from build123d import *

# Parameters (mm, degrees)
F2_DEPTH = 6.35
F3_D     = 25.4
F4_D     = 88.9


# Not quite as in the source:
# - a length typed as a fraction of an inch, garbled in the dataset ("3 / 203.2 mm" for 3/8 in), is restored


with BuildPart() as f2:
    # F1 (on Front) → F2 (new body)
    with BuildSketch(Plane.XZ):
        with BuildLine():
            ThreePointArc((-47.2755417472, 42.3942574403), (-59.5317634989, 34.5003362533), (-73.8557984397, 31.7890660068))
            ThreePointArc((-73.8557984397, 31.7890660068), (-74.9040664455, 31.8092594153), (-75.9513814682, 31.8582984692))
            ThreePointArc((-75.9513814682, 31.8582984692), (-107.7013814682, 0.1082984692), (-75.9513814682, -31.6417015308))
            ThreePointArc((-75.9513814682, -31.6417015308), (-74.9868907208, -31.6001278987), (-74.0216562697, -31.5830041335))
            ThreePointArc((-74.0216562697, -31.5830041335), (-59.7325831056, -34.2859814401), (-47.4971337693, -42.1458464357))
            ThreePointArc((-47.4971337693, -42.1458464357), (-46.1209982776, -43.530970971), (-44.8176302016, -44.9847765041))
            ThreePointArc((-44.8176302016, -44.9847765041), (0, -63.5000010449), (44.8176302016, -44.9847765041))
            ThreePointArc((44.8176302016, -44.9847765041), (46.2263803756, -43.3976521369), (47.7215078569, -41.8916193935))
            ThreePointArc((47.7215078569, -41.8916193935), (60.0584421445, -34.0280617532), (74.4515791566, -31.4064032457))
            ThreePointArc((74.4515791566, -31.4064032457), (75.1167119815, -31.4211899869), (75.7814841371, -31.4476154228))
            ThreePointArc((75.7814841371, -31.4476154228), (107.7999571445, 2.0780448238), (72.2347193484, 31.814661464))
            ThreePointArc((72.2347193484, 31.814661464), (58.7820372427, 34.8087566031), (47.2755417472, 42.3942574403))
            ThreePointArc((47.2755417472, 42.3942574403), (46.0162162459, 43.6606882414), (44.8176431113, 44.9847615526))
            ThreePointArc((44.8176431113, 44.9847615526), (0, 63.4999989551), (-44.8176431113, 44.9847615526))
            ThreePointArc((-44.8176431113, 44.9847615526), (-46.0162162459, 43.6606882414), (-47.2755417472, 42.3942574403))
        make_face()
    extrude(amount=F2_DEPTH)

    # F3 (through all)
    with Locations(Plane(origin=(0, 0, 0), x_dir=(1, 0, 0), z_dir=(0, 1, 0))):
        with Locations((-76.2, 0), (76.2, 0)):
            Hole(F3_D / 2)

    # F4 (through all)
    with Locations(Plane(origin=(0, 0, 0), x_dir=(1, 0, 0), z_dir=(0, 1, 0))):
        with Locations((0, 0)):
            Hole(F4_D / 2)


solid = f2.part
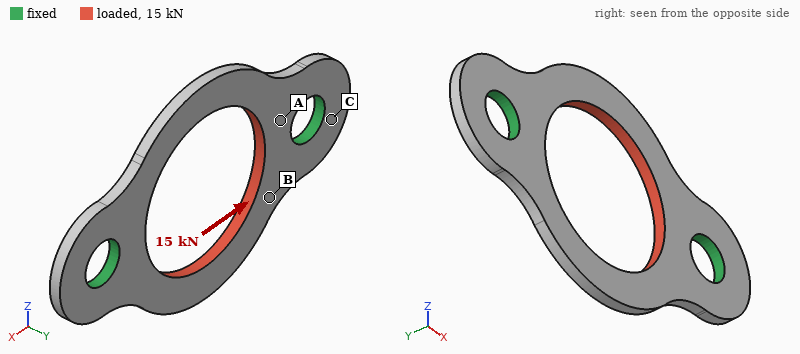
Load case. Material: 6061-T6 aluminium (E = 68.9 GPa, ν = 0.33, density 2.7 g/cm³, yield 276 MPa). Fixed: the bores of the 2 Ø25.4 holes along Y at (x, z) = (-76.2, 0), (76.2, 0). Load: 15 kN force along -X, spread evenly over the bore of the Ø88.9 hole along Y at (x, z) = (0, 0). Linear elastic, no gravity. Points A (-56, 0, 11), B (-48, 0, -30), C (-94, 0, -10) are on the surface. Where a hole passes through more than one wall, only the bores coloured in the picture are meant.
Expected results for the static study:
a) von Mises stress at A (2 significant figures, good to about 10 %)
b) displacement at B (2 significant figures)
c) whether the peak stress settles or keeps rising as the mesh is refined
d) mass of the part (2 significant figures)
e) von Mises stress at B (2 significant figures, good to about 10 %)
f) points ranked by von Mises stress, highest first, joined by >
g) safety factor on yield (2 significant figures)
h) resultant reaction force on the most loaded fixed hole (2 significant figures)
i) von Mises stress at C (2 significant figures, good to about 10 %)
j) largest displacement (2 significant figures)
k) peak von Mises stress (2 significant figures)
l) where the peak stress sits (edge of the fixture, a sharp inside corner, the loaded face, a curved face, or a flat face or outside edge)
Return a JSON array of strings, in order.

["17 MPa", "19 µm", "settles", "180 g", "27 MPa", "B > A > C", "5.7", "7.5 kN", "8.3 MPa", "40 µm", "49 MPa", "the loaded face"]
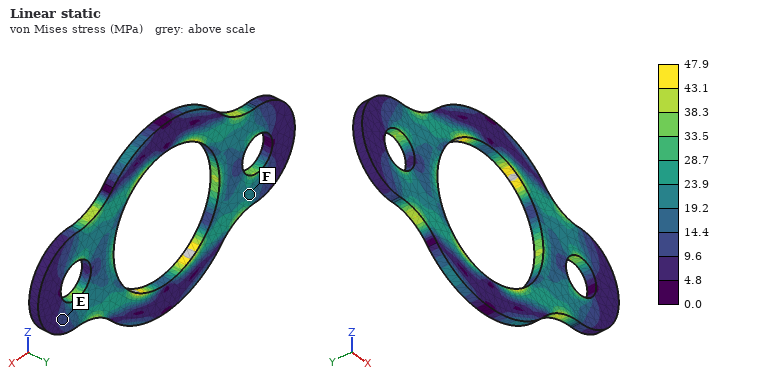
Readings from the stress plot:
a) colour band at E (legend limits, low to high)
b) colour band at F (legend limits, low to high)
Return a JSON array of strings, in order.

["9.6 to 14.4 MPa", "19.2 to 23.9 MPa"]
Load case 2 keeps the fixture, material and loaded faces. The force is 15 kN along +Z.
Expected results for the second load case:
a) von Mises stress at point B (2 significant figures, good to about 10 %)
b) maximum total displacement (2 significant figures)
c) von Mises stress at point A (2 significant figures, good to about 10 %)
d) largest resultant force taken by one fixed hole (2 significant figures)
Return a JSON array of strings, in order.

["24 MPa", "47 µm", "36 MPa", "7.5 kN"]
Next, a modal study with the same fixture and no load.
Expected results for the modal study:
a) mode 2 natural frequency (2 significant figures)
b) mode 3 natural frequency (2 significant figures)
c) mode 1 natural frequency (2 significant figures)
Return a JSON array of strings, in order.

["1200 Hz", "3200 Hz", "1200 Hz"]
